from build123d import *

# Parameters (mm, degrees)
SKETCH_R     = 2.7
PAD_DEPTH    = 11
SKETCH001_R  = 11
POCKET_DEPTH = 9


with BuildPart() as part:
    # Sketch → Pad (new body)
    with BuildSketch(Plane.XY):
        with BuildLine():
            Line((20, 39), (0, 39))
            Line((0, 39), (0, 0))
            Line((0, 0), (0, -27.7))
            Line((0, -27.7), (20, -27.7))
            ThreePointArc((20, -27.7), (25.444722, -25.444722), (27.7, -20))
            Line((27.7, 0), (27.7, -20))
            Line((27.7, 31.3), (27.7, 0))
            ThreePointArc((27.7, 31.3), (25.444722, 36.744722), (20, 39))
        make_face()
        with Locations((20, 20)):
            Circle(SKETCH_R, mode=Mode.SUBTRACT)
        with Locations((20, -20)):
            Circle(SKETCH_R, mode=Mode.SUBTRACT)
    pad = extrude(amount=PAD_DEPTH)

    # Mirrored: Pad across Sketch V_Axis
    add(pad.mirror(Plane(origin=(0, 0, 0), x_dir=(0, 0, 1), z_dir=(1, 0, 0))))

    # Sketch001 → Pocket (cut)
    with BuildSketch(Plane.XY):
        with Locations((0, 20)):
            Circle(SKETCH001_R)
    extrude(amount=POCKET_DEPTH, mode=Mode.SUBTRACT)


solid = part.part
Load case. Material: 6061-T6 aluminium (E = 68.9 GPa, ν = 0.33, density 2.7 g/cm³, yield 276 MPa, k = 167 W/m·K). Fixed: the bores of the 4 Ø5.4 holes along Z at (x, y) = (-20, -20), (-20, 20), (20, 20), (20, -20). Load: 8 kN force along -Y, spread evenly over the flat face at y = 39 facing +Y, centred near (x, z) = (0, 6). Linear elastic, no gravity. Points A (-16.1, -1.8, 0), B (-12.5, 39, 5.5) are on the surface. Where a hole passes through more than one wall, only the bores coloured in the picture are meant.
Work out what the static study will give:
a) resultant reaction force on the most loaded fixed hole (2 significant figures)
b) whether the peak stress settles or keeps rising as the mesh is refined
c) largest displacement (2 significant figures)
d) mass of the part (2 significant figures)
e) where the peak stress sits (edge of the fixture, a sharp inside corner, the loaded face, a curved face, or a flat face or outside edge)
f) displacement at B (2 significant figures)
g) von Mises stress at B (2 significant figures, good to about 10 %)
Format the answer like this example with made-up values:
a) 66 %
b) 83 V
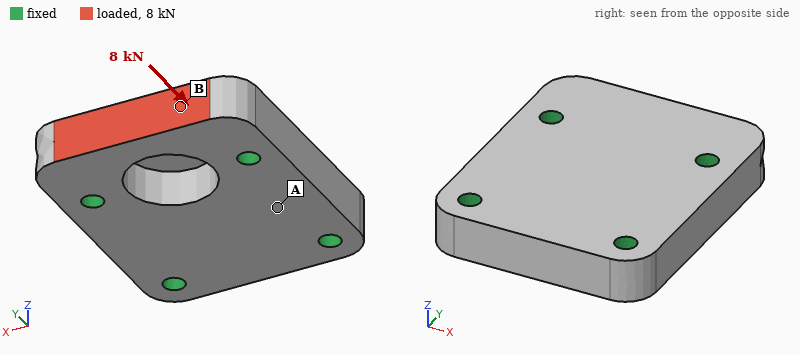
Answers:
a) 3.8 kN
b) keeps rising
c) 17 µm
d) 96 g
e) edge of the fixture
f) 9.0 µm
g) 17 MPa
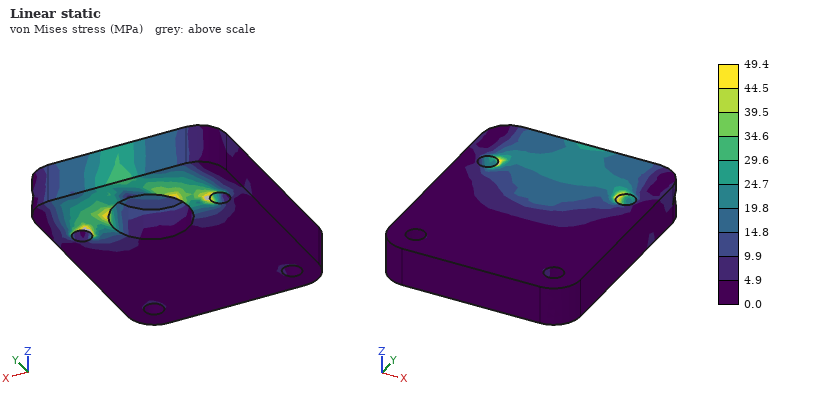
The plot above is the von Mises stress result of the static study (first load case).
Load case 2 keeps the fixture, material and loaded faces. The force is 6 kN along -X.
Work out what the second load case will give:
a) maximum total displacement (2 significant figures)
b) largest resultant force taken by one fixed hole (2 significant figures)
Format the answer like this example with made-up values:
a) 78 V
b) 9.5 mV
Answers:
a) 16 µm
b) 3.8 kN
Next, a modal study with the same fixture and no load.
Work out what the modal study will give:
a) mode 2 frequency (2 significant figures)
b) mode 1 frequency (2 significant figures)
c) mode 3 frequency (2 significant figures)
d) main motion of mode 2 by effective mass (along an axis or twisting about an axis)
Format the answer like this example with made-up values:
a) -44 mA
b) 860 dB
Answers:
a) 19 kHz
b) 16 kHz
c) 25 kHz
d) along Z
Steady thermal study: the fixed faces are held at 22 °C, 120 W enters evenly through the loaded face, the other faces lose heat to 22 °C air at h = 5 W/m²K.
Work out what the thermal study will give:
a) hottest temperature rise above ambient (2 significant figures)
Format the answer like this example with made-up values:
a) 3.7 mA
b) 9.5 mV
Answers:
a) 41 K
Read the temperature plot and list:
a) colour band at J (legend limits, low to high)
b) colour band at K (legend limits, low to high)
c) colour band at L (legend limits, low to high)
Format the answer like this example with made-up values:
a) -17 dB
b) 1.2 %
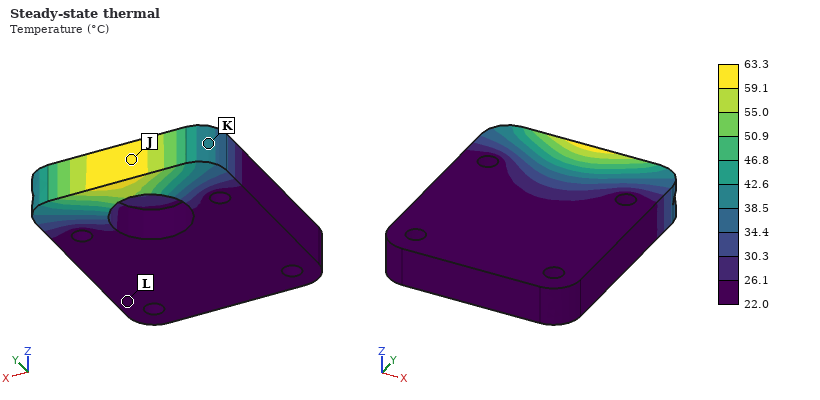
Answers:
a) 59.1 to 63.3 °C
b) 38.5 to 42.6 °C
c) 22.0 to 26.1 °C
